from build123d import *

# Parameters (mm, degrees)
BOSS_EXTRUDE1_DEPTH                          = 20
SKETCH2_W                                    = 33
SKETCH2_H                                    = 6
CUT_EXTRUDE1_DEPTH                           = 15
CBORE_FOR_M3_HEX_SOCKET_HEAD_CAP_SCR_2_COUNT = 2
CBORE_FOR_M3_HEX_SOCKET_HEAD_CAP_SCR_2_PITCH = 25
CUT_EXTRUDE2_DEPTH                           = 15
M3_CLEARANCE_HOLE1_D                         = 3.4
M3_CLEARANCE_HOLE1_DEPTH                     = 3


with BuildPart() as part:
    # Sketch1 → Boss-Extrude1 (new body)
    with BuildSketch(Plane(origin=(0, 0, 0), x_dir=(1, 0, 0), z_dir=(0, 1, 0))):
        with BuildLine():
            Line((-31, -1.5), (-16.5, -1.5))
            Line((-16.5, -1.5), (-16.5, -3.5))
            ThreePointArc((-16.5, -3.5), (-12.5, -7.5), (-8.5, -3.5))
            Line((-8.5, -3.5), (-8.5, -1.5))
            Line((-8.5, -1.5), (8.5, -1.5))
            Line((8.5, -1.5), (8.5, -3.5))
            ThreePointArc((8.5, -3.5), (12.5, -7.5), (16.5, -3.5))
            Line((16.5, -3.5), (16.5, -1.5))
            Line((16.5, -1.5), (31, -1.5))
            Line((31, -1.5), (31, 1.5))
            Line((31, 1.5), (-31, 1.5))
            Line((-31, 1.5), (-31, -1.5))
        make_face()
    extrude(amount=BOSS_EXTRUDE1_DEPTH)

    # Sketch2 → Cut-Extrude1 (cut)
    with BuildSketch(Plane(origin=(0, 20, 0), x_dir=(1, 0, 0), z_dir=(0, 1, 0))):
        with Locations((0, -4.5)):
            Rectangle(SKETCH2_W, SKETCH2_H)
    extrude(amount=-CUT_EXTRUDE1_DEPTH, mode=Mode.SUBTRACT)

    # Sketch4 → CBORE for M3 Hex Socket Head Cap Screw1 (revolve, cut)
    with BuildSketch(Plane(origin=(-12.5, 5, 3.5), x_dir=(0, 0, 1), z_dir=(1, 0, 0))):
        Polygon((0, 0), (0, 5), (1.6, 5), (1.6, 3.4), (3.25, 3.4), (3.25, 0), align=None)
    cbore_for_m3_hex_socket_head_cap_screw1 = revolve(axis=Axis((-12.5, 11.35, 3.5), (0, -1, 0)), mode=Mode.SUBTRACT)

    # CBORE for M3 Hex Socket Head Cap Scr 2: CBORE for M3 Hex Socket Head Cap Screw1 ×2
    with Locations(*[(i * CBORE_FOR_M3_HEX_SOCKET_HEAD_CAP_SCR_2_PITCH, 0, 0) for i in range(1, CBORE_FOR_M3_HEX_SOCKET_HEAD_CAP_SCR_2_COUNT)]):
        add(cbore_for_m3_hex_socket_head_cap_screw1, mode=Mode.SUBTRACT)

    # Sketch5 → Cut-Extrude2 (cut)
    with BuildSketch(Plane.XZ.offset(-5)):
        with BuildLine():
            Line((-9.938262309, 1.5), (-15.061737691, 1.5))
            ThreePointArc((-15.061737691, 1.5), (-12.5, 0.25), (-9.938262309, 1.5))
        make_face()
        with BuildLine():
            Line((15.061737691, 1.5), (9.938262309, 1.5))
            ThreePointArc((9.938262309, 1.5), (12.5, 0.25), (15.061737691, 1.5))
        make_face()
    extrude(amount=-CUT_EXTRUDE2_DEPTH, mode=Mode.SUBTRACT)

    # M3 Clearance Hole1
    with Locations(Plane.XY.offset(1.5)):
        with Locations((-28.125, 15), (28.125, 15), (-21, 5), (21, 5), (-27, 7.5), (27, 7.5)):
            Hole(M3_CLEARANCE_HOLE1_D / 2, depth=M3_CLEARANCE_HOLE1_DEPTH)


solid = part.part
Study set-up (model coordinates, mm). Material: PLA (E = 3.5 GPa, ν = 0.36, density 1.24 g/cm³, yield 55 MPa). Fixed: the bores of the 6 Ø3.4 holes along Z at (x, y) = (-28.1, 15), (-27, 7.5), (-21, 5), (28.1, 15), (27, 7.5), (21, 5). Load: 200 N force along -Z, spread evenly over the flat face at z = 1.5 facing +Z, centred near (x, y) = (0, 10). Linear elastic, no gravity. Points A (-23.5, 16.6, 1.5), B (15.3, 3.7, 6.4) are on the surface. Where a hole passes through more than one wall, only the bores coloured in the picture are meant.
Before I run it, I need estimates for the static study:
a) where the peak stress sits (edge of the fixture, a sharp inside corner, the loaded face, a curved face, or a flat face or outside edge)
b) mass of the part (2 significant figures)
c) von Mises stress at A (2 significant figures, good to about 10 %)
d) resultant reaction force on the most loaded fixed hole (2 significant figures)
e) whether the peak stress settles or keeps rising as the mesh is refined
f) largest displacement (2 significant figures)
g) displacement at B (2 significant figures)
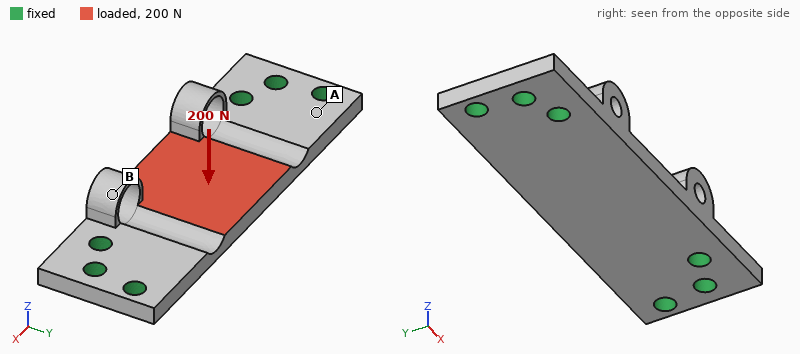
edge of the fixture
4.4 g
17 MPa
110 N
keeps rising
0.72 mm
0.18 mm
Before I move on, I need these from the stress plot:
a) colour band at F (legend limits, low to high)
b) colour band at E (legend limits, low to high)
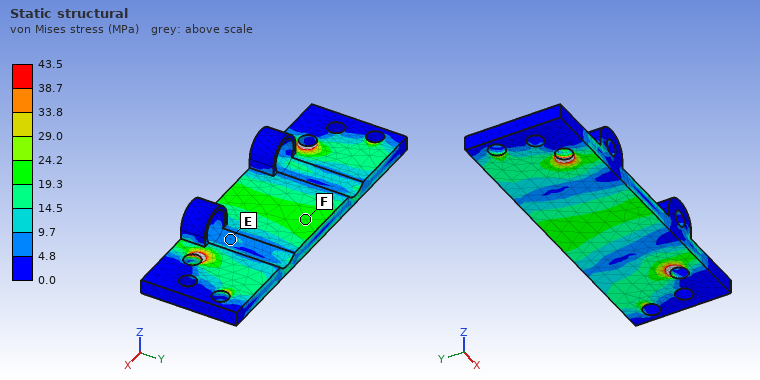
19.3 to 24.2 MPa
4.8 to 9.7 MPa
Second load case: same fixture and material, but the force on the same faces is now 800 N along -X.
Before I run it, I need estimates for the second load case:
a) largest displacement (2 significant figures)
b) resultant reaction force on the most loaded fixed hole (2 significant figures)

0.14 mm
230 N
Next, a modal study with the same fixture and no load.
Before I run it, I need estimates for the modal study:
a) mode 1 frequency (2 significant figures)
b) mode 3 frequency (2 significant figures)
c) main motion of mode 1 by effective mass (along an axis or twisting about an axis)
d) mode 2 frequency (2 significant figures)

2500 Hz
5700 Hz
along Z
3600 Hz
